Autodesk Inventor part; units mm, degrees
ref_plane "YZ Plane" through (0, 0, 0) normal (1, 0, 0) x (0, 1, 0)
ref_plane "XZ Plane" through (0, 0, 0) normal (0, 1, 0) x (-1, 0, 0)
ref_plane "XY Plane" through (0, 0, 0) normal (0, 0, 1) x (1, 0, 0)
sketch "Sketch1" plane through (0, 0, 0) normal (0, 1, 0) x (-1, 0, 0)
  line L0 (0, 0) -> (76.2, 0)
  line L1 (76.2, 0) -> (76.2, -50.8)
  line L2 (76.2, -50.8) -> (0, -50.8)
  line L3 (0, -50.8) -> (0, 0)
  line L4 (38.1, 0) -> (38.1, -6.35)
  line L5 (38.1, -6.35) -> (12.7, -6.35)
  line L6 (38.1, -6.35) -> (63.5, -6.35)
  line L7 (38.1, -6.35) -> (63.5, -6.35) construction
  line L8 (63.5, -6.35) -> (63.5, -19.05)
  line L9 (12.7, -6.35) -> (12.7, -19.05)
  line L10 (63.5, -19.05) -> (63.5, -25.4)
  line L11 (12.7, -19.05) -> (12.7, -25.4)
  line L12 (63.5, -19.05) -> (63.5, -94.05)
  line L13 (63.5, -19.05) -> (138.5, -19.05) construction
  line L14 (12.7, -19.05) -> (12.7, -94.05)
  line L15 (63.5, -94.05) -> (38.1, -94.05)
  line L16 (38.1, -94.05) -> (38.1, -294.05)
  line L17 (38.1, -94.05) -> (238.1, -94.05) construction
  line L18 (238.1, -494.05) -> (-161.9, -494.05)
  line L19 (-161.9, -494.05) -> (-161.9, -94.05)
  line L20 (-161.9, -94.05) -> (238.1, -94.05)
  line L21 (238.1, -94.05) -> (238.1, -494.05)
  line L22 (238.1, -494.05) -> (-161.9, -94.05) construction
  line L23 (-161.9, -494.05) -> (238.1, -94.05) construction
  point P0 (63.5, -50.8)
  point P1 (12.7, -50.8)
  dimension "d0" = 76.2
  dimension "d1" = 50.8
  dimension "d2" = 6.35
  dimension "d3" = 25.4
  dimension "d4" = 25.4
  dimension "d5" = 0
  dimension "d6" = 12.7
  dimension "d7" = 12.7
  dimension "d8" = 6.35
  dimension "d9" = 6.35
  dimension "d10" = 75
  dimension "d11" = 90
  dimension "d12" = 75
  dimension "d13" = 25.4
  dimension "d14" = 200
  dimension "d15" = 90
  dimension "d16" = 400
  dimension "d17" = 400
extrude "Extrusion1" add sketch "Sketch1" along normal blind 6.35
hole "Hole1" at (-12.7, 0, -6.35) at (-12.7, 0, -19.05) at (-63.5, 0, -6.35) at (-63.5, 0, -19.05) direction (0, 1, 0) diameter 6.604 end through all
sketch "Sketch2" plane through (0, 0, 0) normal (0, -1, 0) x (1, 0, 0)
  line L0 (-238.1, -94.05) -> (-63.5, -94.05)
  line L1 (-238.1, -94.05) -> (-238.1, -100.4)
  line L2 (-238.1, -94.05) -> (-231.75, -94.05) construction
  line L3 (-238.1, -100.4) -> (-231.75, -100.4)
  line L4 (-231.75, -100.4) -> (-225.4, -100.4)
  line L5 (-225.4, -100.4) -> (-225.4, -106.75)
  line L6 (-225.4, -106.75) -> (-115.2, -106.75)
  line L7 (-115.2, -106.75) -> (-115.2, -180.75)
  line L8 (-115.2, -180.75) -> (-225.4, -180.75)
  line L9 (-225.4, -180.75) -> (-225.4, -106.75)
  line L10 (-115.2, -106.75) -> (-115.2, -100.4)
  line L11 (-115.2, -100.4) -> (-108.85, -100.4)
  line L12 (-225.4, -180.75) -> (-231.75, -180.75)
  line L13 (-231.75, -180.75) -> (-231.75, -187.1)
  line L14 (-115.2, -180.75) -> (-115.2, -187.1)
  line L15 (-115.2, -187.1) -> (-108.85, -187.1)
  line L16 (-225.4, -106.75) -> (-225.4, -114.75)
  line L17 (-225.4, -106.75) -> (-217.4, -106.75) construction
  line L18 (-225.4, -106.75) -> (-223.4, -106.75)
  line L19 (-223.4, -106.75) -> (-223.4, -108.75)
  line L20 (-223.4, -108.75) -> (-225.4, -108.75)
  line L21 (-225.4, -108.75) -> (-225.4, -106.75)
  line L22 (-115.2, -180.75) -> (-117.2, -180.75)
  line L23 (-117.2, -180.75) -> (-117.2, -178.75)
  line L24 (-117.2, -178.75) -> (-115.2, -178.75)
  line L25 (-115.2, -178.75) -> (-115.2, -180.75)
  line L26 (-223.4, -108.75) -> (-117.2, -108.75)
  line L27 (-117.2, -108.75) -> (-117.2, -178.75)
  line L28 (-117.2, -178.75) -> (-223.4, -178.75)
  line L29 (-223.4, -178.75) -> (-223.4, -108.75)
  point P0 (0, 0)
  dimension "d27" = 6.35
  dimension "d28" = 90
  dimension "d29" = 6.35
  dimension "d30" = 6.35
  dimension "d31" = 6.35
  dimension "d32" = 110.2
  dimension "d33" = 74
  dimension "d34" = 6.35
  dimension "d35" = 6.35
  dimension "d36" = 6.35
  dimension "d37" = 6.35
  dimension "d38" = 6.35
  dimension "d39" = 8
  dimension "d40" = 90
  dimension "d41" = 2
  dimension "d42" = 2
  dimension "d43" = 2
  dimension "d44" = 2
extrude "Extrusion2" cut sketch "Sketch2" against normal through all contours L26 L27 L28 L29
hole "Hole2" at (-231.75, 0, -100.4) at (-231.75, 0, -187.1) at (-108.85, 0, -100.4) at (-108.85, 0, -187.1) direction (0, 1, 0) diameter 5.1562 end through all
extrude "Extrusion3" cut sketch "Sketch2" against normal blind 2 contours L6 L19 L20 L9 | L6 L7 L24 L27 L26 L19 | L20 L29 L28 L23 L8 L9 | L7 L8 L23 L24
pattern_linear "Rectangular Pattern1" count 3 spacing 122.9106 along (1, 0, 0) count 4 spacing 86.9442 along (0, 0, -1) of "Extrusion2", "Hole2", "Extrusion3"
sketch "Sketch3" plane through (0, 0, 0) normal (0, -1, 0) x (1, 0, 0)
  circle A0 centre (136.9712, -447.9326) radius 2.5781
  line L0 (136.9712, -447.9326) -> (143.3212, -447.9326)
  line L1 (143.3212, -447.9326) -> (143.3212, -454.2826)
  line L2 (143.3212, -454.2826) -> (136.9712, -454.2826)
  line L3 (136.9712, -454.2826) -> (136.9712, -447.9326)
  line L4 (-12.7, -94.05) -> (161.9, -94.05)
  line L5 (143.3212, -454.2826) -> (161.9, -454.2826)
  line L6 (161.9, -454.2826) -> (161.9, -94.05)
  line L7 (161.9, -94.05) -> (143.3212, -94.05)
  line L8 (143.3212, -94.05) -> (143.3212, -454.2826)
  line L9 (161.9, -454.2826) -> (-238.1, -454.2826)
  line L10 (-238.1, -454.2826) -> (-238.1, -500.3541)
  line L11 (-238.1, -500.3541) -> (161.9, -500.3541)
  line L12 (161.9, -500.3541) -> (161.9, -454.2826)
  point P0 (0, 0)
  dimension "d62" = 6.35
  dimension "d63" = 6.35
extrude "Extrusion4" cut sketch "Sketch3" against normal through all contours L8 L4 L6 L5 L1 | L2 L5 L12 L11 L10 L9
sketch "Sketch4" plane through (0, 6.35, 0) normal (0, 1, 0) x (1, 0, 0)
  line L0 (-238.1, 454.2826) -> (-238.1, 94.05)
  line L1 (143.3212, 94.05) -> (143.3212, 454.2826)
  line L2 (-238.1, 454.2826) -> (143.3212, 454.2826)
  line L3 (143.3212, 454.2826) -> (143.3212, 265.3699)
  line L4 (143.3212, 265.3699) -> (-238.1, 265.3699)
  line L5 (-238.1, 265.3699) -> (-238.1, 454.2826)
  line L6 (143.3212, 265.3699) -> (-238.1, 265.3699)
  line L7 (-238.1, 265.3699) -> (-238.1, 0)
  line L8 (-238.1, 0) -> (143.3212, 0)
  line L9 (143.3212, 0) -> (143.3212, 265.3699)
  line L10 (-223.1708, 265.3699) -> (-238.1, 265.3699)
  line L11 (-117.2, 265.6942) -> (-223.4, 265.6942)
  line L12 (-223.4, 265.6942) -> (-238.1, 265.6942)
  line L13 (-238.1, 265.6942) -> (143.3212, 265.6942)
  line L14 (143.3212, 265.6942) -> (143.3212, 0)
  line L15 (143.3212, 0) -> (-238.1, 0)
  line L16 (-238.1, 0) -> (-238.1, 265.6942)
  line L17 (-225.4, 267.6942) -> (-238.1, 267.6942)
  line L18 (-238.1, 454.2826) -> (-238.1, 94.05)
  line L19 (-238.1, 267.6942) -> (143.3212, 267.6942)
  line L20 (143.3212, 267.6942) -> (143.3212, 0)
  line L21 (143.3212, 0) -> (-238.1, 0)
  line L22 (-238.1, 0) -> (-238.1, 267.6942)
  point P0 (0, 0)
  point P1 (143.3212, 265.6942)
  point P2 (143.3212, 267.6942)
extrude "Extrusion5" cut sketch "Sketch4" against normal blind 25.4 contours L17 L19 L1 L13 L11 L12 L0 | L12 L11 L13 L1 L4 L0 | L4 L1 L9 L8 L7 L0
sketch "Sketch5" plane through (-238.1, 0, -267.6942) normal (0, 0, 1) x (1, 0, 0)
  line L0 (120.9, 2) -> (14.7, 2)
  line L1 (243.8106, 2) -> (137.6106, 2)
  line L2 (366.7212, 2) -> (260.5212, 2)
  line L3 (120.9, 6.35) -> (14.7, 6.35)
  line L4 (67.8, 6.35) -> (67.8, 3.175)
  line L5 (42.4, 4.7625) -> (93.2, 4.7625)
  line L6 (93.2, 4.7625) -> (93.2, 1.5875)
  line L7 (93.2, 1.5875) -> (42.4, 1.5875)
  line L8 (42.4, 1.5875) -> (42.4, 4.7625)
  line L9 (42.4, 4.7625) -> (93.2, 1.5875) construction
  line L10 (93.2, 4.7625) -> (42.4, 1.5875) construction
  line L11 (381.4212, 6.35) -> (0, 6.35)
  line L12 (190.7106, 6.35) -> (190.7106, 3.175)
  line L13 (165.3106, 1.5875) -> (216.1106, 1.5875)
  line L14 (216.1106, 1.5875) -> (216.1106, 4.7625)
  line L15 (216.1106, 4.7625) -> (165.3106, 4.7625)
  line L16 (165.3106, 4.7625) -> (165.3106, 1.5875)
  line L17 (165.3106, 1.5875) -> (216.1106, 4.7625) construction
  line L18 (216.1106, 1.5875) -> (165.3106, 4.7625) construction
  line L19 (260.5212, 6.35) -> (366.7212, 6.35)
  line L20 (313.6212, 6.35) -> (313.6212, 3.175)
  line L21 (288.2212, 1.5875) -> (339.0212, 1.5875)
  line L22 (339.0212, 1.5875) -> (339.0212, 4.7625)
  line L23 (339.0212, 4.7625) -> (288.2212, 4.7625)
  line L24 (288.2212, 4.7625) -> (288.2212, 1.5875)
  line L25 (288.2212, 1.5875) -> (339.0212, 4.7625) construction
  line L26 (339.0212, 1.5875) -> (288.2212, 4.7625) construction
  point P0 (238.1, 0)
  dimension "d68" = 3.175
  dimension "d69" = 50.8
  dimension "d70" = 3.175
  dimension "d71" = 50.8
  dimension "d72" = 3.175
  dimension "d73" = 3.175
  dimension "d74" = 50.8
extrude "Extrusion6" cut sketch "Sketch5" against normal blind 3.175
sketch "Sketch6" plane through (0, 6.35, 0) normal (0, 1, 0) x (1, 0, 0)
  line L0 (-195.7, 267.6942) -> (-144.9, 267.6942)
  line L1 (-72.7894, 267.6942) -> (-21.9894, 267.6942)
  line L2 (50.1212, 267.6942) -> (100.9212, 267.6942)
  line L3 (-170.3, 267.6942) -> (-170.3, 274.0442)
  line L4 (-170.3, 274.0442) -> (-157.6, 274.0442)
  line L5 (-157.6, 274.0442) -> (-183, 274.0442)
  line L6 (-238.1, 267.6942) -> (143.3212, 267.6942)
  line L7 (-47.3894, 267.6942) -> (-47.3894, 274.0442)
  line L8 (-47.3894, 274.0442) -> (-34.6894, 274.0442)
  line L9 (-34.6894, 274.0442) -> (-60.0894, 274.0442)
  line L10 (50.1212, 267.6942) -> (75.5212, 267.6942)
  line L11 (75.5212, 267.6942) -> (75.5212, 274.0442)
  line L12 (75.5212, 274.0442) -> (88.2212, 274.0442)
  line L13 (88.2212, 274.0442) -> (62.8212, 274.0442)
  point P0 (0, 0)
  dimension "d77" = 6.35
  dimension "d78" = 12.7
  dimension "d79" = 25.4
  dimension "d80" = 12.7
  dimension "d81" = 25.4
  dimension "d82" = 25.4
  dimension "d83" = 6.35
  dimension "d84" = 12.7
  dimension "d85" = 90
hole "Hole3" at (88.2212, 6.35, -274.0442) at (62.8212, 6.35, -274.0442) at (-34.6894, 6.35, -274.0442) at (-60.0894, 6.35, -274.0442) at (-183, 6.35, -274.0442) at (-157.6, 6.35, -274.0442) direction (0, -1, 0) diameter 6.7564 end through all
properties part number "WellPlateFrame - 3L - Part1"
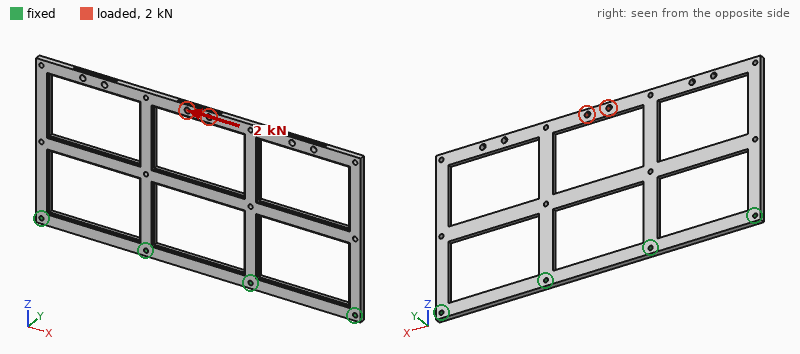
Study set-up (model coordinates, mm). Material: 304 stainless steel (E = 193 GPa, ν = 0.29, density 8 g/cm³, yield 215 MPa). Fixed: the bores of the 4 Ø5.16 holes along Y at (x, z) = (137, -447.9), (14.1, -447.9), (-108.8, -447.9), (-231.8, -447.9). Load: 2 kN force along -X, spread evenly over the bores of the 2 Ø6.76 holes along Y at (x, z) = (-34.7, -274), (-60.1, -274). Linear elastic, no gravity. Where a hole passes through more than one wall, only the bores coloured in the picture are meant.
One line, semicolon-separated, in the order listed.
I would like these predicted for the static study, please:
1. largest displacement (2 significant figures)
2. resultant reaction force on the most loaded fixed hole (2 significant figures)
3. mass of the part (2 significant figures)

0.32 mm; 880 N; 1.2 kg
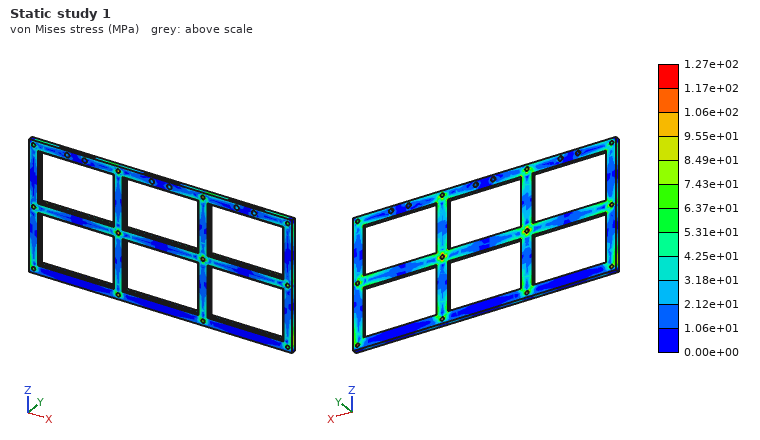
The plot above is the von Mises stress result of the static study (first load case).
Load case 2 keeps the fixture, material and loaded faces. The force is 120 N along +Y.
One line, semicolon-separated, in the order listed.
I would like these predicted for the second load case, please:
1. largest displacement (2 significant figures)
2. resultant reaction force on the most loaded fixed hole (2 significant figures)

1.1 mm; 51 N
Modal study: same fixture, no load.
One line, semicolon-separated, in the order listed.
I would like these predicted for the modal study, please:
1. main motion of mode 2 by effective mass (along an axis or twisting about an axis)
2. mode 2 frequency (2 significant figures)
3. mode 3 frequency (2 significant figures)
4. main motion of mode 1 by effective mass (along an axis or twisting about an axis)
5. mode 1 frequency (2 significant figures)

twisting about Z; 160 Hz; 300 Hz; along Y; 96 Hz
